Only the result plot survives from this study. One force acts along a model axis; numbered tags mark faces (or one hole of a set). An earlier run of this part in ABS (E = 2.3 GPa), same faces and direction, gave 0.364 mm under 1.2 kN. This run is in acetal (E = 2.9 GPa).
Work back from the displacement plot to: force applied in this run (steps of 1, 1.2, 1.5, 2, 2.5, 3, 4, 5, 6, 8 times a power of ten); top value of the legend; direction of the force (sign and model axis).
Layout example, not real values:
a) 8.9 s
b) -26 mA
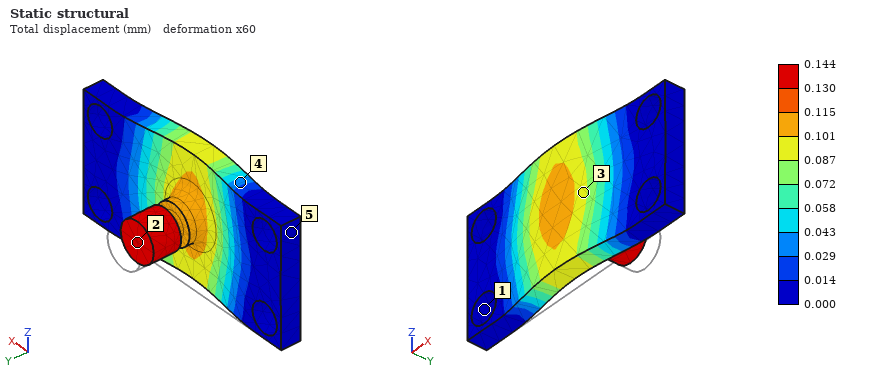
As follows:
a) 600 N
b) 0.144 mm
c) -Y
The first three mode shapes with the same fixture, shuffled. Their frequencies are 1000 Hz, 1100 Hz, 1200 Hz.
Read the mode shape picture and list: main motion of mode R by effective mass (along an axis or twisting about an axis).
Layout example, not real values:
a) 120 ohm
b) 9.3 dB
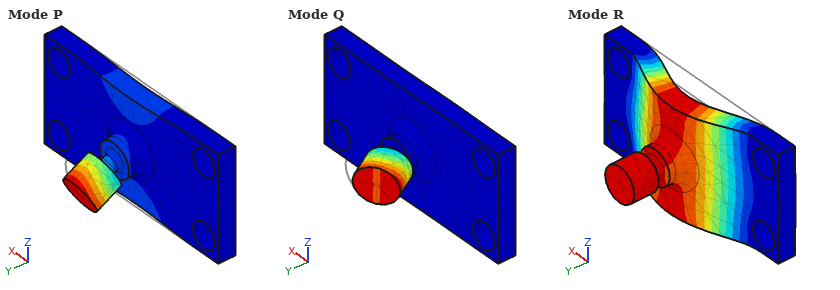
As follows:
a) along Y
